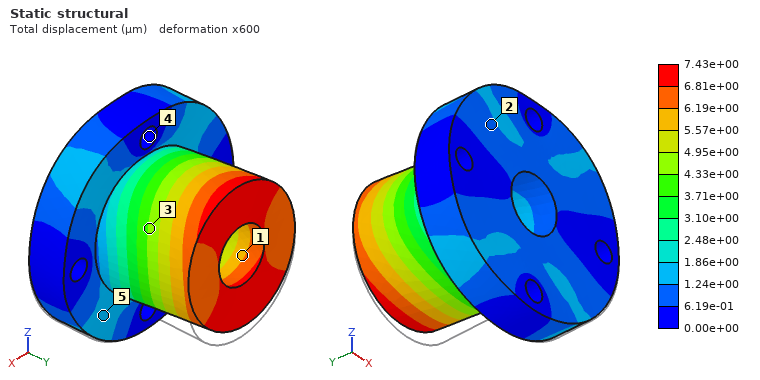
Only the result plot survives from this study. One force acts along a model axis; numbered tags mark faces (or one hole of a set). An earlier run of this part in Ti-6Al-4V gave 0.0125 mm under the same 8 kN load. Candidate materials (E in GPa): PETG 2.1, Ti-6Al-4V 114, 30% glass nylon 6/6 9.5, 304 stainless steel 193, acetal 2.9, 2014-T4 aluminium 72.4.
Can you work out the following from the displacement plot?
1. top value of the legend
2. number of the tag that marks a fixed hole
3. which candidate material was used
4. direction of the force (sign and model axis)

7.43e+00 µm
4
304 stainless steel
+Z
